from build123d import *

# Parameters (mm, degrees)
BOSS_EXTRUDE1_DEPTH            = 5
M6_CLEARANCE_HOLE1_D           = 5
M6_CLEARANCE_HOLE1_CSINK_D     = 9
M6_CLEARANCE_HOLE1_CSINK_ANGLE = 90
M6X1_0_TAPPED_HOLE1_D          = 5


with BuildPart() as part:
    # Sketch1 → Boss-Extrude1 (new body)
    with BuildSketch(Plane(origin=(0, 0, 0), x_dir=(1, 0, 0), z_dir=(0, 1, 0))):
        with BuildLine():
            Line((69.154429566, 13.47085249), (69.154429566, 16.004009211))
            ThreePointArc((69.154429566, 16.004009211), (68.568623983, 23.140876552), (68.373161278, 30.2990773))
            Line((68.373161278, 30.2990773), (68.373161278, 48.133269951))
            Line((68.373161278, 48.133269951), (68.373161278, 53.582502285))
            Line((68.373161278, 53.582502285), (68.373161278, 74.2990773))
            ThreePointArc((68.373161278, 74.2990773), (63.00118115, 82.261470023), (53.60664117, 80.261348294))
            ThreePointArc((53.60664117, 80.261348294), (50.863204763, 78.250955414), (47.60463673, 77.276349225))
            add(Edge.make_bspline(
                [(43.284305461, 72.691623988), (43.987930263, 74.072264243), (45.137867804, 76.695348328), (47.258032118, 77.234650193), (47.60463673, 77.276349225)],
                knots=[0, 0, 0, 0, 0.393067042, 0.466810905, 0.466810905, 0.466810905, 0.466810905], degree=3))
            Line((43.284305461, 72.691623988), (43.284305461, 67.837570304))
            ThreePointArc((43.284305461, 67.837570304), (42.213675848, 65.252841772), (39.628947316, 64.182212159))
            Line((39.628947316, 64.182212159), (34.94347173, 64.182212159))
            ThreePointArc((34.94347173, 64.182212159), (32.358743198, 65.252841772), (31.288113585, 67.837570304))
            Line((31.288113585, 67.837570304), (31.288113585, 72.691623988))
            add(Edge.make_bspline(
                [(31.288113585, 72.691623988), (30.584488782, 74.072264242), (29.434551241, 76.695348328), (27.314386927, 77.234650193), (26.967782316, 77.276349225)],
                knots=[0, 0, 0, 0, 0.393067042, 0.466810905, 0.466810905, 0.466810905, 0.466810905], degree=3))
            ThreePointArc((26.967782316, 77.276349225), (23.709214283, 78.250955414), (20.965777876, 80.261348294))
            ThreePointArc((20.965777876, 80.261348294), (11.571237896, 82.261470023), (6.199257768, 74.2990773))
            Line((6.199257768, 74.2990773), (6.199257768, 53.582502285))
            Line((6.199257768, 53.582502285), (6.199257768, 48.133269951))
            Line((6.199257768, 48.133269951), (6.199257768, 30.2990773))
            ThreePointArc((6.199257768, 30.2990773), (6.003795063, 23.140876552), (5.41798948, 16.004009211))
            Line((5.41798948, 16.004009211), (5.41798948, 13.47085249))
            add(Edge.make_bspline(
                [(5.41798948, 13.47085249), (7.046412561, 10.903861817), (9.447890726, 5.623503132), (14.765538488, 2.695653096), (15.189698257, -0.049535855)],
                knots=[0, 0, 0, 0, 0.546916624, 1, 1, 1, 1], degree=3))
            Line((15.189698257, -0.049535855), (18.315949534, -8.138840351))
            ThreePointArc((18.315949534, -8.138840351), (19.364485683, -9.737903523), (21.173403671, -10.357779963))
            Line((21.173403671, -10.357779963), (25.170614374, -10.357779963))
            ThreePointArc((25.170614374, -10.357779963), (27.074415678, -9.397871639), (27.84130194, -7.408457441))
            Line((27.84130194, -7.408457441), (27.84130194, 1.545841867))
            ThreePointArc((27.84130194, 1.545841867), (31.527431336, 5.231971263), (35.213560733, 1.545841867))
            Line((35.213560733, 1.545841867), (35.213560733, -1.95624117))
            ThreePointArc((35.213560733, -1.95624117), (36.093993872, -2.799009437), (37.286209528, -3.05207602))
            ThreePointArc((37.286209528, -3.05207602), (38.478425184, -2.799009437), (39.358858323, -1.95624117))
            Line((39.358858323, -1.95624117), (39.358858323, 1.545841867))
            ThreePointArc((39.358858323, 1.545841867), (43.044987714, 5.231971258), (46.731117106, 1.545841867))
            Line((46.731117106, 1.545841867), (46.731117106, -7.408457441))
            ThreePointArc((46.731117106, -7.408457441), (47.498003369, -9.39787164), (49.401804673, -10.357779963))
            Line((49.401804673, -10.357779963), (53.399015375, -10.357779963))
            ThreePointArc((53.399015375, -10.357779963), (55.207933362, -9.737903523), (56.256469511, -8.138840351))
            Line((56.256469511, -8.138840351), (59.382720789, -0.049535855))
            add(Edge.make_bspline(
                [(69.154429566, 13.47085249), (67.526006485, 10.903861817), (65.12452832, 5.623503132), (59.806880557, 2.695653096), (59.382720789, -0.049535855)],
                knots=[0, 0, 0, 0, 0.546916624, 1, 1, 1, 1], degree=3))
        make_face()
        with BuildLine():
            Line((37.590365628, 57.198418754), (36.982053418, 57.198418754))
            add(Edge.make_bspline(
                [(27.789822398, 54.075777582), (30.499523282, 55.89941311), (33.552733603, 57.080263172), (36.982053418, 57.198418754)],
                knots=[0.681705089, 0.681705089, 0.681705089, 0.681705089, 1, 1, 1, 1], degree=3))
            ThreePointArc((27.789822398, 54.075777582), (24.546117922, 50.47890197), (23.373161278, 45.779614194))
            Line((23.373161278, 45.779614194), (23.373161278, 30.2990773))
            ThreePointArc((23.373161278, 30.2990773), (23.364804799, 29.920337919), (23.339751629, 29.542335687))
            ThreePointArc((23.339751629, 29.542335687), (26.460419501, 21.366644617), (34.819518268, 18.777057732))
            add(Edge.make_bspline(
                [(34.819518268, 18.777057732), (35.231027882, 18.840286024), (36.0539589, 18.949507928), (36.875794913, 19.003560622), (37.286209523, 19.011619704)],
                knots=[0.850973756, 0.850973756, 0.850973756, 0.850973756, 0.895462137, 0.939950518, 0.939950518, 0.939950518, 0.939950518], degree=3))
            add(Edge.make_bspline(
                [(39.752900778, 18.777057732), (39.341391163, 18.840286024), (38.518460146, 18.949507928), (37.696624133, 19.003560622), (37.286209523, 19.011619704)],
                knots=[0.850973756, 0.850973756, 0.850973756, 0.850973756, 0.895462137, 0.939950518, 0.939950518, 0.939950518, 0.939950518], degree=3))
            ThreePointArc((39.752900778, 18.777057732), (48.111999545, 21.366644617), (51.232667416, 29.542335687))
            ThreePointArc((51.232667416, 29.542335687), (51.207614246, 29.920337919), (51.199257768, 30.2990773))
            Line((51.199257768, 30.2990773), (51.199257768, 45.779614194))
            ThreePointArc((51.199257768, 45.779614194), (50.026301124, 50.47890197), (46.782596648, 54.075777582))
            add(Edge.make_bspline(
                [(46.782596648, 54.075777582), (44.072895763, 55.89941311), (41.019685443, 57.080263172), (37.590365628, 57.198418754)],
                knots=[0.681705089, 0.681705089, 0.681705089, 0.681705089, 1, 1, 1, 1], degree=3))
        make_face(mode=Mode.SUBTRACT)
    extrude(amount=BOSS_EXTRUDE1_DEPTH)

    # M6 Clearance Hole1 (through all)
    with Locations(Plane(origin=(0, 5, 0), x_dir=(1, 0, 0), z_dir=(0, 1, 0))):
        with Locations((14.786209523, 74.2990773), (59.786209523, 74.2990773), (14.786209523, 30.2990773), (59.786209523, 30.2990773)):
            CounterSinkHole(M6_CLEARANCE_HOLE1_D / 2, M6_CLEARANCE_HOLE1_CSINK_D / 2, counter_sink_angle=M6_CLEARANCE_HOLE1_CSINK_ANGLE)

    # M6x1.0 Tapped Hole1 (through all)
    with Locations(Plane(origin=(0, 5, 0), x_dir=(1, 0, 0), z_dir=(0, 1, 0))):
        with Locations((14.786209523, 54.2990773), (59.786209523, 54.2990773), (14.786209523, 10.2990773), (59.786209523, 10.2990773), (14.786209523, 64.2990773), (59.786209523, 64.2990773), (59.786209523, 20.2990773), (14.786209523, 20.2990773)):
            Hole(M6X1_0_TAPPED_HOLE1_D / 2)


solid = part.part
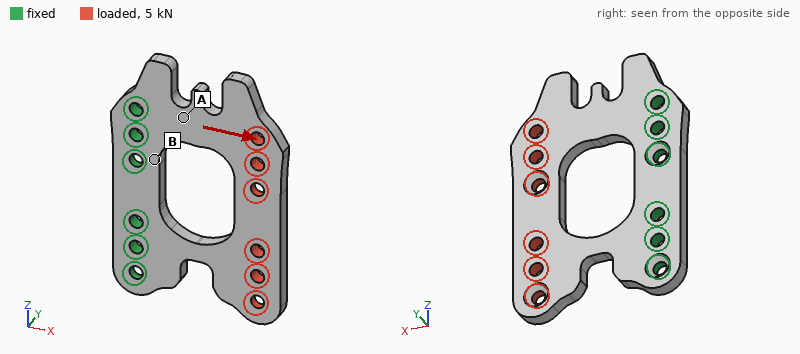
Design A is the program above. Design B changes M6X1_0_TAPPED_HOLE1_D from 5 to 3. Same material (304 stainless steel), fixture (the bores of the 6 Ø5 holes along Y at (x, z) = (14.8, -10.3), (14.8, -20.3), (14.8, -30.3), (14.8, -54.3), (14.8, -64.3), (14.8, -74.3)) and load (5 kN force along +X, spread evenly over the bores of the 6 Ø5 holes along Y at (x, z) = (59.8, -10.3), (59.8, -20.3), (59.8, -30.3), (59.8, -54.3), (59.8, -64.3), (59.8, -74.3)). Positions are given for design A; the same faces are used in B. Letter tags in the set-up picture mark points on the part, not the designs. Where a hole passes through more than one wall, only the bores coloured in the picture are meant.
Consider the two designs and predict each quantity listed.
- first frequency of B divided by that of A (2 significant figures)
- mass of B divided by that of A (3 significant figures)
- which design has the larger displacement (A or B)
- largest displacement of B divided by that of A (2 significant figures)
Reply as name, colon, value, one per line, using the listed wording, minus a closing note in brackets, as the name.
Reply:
first frequency of B divided by that of A: 0.96
mass of B divided by that of A: 1.03
which design has the larger displacement: B
largest displacement of B divided by that of A: 1.4
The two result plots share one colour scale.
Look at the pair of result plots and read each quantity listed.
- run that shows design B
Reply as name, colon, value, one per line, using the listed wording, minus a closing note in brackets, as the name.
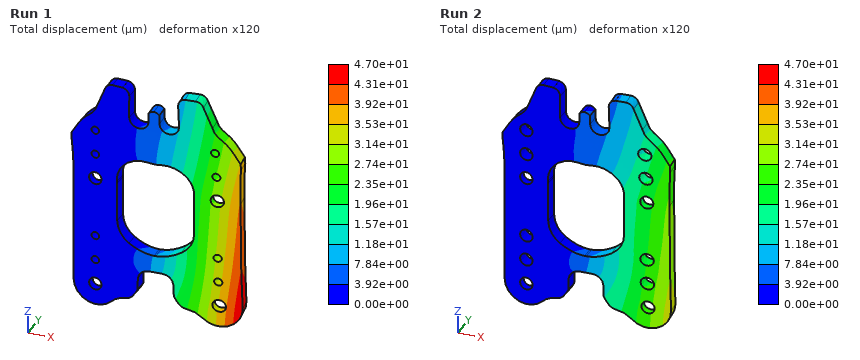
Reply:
run that shows design B: Run 1
